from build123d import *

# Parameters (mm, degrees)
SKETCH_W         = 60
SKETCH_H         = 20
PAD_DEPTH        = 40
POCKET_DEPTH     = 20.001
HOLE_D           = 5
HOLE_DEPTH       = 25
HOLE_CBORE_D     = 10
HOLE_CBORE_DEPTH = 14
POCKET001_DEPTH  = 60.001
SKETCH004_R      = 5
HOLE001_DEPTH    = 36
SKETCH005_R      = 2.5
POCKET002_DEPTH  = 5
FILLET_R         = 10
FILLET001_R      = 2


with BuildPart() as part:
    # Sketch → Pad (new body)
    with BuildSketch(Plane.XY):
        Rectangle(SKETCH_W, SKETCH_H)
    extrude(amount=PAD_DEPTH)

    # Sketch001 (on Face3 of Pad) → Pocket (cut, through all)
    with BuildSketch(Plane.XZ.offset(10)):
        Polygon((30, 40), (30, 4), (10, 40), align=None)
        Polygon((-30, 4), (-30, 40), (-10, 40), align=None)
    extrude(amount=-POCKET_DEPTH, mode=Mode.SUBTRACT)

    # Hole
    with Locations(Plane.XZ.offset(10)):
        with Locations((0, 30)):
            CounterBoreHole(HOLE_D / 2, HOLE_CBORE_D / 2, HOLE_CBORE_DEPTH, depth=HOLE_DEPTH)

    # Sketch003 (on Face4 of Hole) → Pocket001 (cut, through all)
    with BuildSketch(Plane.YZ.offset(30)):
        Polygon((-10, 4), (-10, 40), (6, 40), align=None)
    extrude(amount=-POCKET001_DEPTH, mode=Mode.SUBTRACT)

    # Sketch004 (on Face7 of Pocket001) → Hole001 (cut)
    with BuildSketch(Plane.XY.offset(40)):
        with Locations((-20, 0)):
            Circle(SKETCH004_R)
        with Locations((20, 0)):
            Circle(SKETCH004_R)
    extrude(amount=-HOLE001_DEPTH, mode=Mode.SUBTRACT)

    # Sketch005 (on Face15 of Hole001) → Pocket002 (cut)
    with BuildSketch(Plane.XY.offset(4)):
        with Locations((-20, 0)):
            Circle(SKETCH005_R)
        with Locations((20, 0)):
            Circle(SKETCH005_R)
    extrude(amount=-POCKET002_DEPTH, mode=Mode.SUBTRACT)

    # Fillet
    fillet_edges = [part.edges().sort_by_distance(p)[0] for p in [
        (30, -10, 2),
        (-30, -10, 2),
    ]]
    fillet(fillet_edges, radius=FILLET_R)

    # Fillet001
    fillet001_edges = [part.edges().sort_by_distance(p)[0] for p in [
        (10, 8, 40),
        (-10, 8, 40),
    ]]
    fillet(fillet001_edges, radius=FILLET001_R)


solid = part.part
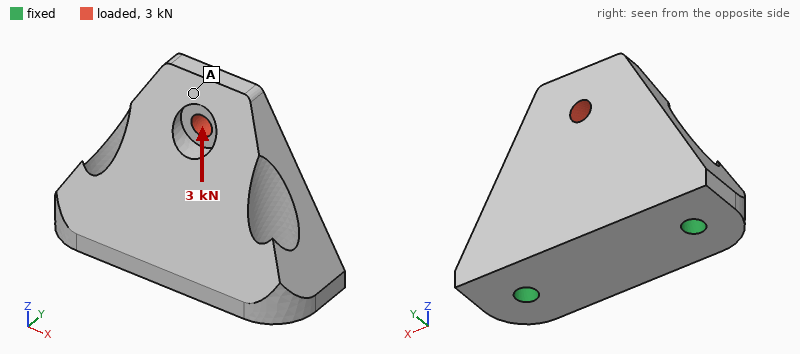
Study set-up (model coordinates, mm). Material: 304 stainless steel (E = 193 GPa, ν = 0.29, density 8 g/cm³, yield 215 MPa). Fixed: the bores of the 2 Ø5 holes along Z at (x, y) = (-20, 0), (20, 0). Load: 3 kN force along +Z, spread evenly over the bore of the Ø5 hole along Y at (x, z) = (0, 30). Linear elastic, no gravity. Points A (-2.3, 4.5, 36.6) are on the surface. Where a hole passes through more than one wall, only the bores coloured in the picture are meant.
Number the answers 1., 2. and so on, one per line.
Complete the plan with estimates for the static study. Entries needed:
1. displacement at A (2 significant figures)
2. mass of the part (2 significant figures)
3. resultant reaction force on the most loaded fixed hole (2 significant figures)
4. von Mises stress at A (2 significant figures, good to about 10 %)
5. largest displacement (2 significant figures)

1. 29 µm
2. 170 g
3. 1.6 kN
4. 28 MPa
5. 34 µm
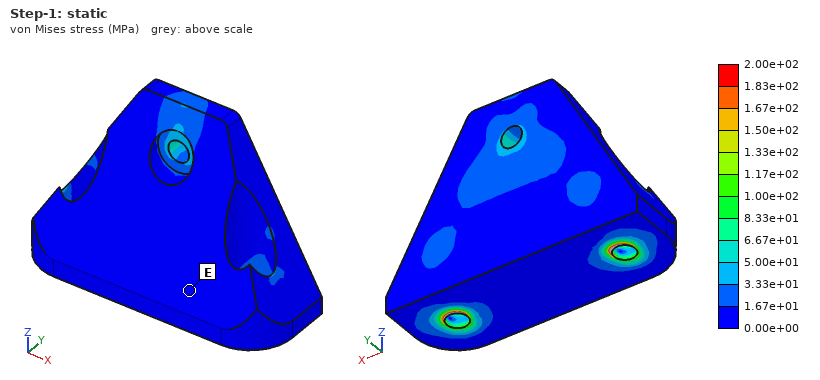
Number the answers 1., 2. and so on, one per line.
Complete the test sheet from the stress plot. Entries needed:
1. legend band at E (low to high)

1. 0.00e+00 to 1.67e+01 MPa
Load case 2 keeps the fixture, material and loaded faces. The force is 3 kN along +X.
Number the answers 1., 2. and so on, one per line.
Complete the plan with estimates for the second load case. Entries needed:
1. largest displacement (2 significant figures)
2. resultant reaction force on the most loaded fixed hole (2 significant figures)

1. 9.8 µm
2. 2.6 kN
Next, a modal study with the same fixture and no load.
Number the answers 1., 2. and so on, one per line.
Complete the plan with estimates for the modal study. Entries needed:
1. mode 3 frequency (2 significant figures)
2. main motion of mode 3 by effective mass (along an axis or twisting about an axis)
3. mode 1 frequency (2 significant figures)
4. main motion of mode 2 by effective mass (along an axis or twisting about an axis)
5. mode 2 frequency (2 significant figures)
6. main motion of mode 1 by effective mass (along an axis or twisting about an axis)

1. 15 kHz
2. along Z
3. 4000 Hz
4. along X
5. 14 kHz
6. along Y
